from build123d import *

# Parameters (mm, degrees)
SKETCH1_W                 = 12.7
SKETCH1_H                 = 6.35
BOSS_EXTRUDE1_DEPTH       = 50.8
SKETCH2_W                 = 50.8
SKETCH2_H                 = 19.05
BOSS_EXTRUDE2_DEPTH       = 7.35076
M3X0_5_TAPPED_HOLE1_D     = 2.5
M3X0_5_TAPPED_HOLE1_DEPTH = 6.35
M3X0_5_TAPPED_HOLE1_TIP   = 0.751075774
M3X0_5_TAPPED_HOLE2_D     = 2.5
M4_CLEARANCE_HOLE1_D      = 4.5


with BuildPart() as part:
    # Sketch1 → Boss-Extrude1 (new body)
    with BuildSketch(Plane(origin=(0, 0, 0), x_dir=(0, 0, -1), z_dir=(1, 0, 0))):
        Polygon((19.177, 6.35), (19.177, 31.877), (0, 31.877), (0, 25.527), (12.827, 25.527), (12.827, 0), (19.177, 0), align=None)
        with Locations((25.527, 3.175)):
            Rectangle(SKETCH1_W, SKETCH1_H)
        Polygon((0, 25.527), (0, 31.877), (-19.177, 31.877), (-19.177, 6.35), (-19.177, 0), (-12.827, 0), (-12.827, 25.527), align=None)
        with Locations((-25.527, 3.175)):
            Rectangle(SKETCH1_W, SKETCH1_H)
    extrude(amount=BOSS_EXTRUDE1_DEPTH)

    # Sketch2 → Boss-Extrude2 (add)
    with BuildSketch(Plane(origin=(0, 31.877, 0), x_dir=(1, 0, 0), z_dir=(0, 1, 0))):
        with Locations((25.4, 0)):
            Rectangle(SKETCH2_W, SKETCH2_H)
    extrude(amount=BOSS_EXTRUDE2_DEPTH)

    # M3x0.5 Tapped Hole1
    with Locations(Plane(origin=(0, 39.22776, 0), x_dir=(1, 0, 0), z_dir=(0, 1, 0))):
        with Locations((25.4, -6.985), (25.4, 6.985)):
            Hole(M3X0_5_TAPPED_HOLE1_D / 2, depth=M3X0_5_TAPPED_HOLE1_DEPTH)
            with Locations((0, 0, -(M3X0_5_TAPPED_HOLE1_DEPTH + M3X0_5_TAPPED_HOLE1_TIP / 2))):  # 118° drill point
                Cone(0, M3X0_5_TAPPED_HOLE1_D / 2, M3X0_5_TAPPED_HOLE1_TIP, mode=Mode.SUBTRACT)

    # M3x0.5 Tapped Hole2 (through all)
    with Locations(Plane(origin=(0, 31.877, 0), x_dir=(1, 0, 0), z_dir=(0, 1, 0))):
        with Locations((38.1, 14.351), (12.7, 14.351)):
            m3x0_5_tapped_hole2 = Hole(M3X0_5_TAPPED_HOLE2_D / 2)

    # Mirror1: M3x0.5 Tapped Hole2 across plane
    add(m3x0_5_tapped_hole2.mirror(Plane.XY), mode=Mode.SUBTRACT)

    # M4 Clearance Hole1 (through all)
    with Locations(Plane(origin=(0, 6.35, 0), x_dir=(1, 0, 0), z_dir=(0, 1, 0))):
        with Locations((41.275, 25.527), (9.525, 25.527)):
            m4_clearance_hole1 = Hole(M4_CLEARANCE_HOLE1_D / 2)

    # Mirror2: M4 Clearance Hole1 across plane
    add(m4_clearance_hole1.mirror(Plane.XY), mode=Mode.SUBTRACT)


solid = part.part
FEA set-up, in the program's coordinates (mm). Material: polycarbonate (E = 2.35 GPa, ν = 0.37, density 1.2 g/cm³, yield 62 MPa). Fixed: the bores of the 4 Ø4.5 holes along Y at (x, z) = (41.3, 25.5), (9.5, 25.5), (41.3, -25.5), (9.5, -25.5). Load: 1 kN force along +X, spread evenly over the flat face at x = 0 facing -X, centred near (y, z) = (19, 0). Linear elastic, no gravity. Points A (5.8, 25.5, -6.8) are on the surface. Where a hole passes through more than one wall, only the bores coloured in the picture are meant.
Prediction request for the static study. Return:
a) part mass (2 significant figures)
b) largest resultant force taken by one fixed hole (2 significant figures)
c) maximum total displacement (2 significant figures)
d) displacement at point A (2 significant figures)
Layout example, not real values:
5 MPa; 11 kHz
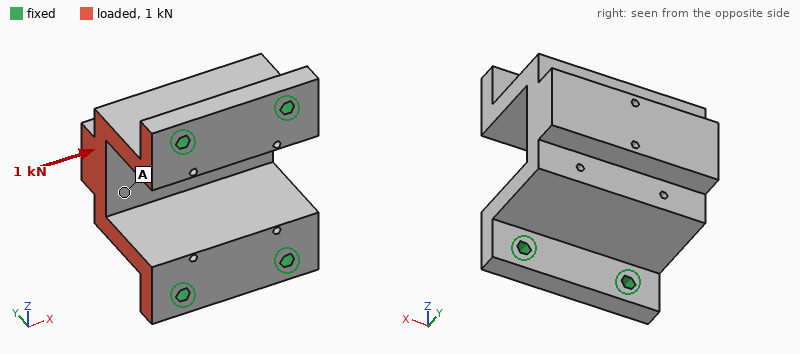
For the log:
52 g; 400 N; 0.20 mm; 0.14 mm
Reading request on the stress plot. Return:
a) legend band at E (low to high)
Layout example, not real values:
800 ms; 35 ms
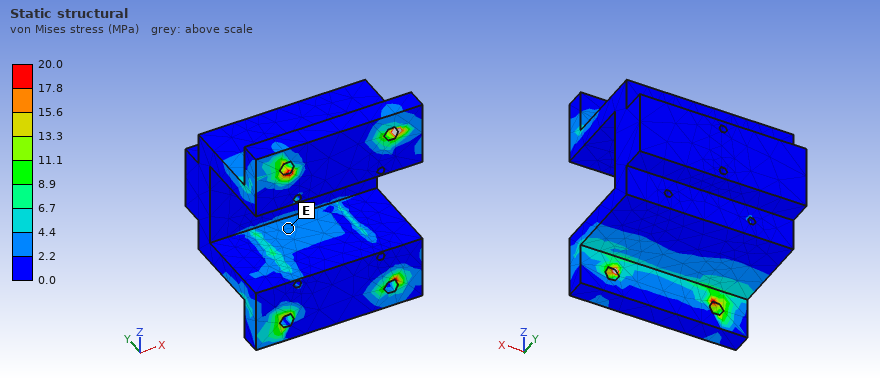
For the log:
2.2 to 4.4 MPa
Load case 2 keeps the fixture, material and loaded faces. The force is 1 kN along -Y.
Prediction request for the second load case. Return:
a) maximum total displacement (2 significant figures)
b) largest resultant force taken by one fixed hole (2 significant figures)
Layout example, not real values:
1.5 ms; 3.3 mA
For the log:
0.31 mm; 610 N
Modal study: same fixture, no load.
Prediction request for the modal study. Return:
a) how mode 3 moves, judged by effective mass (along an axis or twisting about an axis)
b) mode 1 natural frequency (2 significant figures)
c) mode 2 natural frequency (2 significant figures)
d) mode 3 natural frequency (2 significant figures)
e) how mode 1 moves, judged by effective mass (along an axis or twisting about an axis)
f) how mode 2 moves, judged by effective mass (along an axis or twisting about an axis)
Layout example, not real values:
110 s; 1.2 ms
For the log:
twisting about Y; 1400 Hz; 1800 Hz; 2300 Hz; along Z; along X
